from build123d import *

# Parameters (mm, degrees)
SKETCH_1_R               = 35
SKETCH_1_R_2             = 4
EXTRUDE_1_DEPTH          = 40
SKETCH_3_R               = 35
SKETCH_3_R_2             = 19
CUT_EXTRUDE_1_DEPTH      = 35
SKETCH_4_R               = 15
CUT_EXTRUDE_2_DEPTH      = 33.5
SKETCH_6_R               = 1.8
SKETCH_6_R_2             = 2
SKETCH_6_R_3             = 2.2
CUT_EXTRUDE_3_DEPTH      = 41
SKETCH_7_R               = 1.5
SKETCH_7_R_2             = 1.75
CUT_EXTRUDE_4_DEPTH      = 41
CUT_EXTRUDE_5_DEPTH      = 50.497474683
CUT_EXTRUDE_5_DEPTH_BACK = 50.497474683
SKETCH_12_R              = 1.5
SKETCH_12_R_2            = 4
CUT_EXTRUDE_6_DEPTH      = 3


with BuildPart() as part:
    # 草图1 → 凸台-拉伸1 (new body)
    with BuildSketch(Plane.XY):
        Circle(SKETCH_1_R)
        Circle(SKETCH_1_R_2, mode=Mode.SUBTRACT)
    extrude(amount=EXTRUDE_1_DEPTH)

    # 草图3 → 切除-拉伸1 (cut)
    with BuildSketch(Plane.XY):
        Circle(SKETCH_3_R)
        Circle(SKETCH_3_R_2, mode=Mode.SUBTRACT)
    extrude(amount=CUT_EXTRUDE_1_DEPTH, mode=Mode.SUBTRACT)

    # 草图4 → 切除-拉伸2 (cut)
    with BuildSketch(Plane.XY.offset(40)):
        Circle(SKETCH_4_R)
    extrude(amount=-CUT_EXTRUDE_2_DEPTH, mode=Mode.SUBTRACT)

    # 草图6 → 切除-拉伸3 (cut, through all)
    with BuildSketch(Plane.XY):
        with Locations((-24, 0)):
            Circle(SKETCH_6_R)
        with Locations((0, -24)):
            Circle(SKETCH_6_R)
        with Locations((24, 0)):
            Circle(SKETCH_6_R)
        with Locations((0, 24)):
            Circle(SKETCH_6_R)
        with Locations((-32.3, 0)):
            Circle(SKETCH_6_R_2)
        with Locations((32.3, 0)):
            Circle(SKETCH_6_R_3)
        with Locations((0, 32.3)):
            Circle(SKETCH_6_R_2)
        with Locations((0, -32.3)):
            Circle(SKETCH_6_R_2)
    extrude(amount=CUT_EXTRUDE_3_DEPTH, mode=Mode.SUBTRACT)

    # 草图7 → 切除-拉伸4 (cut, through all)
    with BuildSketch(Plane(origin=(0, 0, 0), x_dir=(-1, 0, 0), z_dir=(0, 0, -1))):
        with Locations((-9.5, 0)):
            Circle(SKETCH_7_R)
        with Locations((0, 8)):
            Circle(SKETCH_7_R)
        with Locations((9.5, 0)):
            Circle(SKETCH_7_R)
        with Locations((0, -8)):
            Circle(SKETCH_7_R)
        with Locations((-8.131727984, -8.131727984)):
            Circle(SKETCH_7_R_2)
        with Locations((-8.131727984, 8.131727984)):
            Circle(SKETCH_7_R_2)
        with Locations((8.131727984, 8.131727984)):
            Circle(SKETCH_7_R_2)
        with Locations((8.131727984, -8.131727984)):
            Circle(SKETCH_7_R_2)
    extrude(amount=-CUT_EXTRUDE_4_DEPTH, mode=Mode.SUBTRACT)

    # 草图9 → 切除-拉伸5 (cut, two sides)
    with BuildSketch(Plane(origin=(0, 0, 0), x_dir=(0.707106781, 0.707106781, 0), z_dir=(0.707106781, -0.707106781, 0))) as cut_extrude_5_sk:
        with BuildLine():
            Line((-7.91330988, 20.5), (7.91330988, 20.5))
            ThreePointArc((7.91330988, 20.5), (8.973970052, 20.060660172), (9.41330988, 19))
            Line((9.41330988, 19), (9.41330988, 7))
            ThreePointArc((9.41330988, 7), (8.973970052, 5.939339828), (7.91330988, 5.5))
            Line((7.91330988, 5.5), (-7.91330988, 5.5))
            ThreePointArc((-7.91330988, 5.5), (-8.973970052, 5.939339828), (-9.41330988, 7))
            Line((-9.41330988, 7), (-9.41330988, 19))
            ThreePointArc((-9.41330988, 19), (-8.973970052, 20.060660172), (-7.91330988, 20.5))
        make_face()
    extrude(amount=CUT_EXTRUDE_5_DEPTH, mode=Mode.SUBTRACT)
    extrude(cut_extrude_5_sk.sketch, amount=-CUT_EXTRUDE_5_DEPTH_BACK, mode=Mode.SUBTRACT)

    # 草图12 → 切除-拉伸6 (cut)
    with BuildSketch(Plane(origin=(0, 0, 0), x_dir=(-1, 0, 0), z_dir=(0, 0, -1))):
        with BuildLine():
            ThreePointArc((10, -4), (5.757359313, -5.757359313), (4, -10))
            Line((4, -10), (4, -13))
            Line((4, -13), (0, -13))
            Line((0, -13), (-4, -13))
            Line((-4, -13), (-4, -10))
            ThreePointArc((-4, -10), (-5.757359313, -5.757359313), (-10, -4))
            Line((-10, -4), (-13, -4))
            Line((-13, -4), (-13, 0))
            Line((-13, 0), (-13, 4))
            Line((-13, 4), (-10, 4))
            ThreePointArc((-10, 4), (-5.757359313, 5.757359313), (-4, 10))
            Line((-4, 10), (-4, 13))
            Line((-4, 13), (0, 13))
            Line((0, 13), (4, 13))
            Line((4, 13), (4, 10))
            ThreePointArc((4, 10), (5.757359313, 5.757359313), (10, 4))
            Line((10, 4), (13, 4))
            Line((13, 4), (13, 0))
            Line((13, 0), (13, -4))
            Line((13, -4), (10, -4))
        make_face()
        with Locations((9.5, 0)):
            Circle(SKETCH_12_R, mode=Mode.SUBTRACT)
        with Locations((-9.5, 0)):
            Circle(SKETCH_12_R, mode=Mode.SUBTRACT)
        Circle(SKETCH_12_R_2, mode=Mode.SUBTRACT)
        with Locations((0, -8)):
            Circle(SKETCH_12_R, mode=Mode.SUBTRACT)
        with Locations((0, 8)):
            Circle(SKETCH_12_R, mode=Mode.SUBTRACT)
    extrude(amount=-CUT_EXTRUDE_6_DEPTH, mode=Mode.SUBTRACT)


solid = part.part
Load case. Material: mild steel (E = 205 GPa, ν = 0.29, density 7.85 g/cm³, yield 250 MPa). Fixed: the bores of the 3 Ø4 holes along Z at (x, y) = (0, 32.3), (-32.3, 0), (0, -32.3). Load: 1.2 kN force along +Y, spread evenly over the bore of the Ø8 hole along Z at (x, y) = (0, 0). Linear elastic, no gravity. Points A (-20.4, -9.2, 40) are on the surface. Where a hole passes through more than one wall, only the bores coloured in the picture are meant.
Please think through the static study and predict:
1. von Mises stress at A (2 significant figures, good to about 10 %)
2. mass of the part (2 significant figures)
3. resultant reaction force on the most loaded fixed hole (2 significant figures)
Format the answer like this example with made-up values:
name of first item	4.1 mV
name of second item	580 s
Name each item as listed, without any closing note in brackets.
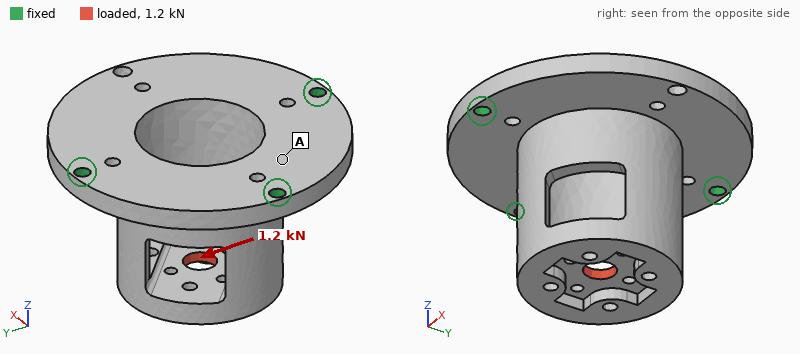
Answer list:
von Mises stress at A	11 MPa
mass of the part	240 g
resultant reaction force on the most loaded fixed hole	890 N
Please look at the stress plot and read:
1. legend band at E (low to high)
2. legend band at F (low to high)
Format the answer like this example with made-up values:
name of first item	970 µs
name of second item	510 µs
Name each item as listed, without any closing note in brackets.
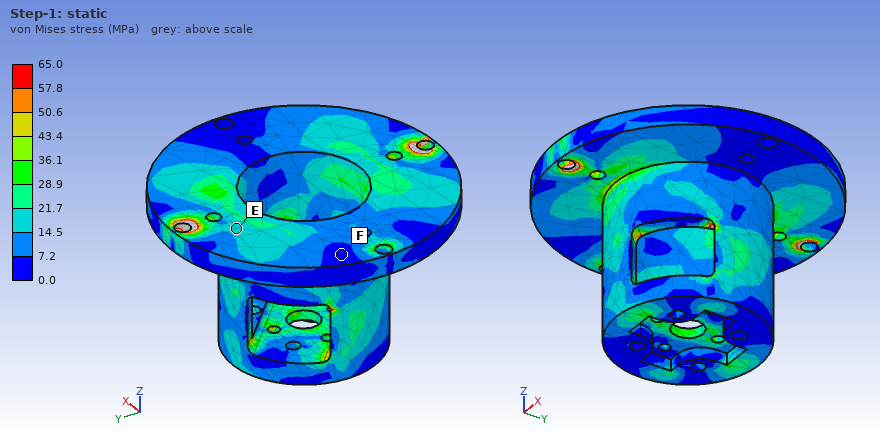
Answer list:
legend band at E	14.5 to 21.7 MPa
legend band at F	0.0 to 7.2 MPa
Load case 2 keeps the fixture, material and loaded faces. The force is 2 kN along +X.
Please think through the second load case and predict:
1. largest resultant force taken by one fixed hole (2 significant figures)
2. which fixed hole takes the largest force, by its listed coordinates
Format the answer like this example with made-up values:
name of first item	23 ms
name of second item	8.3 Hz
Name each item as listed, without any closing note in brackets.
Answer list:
largest resultant force taken by one fixed hole	2.1 kN
which fixed hole takes the largest force, by its listed coordinates	(-32.3, 0)
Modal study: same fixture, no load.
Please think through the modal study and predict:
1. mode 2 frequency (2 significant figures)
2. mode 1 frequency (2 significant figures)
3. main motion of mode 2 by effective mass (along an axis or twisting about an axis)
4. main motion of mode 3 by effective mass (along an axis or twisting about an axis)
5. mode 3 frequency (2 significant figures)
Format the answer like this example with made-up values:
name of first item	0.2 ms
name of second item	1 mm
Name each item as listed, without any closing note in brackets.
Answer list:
mode 2 frequency	4600 Hz
mode 1 frequency	2500 Hz
main motion of mode 2 by effective mass	along Y
main motion of mode 3 by effective mass	along Z
mode 3 frequency	6000 Hz
